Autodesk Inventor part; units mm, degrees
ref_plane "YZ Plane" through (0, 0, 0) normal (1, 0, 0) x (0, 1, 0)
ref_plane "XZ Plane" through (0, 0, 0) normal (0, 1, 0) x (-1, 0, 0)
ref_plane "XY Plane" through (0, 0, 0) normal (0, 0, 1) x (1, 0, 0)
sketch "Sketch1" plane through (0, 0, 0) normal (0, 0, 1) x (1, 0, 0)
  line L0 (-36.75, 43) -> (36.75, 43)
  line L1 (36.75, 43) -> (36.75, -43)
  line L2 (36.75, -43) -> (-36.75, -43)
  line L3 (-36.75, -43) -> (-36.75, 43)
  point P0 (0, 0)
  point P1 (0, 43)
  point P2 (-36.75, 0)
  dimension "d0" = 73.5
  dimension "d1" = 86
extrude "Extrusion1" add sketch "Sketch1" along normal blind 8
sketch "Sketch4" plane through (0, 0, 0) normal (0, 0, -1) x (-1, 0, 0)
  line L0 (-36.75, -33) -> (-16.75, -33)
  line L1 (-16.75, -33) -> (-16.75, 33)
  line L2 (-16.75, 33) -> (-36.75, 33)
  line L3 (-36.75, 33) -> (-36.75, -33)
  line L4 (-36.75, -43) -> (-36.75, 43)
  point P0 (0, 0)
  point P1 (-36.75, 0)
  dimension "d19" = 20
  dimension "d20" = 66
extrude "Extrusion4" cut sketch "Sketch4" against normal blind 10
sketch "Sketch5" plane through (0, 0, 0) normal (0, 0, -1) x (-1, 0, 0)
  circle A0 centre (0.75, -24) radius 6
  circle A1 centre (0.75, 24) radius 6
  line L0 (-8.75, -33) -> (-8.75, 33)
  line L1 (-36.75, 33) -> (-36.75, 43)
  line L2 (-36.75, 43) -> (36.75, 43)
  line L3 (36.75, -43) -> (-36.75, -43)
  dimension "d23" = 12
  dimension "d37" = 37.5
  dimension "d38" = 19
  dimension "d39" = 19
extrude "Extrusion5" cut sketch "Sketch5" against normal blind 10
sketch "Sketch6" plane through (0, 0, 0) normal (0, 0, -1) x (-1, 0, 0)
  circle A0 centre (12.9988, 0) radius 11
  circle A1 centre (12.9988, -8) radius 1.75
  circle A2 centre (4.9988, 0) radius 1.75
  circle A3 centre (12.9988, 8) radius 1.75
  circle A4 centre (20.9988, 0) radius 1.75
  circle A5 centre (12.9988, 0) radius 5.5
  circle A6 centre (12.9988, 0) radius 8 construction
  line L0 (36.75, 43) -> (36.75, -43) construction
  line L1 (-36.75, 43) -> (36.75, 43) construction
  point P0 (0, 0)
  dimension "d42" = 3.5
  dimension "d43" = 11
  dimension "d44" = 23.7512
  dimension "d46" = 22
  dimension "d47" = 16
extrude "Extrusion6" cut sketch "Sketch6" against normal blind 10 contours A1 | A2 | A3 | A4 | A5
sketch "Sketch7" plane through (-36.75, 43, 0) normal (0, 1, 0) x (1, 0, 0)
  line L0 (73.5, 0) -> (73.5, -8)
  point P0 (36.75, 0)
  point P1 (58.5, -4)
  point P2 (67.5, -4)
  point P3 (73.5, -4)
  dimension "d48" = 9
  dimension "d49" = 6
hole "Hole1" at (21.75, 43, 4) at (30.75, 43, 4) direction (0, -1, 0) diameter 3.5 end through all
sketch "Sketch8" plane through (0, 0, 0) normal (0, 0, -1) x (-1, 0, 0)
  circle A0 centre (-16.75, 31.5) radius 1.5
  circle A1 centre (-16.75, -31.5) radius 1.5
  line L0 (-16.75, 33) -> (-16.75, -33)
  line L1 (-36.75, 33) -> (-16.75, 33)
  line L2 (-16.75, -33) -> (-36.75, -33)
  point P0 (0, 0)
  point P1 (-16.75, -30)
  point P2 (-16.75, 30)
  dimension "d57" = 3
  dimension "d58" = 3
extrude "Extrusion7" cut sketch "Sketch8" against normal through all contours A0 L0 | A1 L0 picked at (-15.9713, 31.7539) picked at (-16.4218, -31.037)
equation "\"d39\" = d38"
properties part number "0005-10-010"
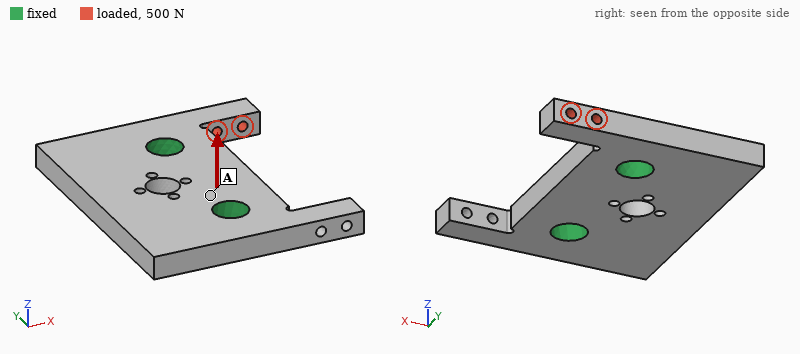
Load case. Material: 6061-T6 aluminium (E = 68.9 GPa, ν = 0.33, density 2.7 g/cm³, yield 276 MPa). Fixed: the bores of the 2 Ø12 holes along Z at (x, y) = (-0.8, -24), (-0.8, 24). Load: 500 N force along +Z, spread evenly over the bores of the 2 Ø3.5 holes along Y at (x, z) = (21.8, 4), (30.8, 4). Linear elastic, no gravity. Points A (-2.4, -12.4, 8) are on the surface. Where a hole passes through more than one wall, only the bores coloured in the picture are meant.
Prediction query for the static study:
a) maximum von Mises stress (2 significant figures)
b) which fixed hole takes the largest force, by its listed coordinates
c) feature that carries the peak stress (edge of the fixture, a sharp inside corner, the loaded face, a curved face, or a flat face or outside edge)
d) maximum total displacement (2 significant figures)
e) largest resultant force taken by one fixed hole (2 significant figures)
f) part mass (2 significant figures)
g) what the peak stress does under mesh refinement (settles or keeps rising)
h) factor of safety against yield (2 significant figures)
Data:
100 MPa
(-0.8, 24)
a curved face
0.11 mm
520 N
99 g
settles
2.7
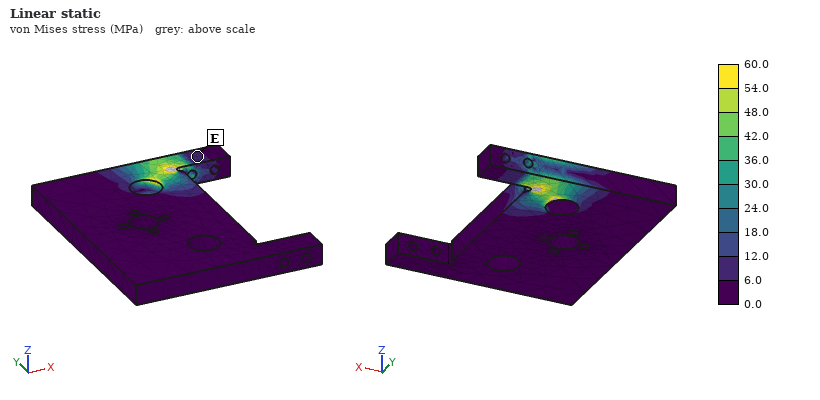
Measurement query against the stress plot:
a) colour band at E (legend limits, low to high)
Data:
6.0 to 12.0 MPa
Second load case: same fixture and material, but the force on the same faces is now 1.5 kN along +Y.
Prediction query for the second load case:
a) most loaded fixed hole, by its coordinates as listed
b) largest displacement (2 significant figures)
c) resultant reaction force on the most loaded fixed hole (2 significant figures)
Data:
(-0.8, 24)
0.13 mm
1.4 kN
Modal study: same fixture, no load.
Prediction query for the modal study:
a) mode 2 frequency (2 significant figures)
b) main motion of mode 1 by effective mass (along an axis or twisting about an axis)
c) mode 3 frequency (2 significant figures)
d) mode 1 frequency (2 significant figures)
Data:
6200 Hz
along Z
6300 Hz
5400 Hz
